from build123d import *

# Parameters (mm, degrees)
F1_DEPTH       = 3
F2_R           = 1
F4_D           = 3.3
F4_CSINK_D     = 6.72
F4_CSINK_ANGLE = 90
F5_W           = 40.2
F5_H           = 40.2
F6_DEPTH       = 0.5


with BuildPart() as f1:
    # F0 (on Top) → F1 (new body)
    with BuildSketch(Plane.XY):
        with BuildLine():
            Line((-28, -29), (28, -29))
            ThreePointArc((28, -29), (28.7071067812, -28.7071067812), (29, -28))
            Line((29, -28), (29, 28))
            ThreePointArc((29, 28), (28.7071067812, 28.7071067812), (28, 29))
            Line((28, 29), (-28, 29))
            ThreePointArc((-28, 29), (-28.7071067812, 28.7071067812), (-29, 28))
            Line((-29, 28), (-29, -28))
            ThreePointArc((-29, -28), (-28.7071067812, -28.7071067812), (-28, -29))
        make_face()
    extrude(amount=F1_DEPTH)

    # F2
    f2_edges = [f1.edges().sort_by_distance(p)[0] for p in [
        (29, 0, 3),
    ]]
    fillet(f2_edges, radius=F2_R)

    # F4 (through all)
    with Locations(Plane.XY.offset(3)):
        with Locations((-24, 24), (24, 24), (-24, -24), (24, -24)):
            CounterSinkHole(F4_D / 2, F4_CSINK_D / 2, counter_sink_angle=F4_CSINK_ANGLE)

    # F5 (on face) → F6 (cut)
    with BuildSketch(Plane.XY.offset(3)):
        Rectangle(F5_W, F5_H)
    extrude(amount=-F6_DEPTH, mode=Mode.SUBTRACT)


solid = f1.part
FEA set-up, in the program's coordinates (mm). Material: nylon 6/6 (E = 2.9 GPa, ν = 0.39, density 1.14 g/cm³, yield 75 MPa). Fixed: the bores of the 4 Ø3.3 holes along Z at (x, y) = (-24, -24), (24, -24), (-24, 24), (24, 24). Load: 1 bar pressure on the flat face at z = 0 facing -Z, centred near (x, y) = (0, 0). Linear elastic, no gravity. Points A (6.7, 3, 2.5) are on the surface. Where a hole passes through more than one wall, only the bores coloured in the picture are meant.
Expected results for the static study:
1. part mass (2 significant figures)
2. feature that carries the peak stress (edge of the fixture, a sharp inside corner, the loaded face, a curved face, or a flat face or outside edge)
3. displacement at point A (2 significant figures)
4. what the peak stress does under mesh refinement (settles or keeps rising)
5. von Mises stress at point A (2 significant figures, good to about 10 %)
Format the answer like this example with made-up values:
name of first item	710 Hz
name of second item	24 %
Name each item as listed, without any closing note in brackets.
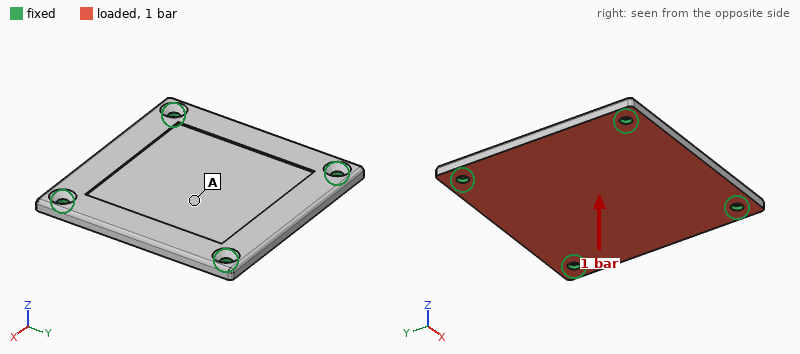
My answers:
part mass	10 g
feature that carries the peak stress	edge of the fixture
displacement at point A	0.84 mm
what the peak stress does under mesh refinement	keeps rising
von Mises stress at point A	12 MPa
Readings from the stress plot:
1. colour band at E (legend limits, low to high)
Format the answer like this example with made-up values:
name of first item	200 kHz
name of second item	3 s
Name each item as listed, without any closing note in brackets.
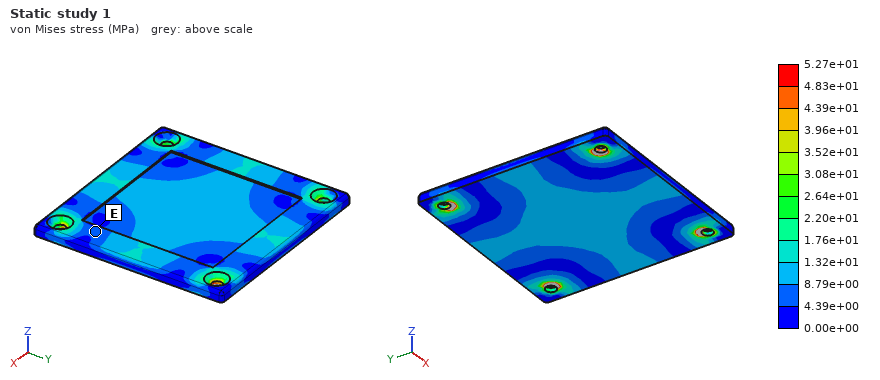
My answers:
colour band at E	4.39e+00 to 8.79e+00 MPa
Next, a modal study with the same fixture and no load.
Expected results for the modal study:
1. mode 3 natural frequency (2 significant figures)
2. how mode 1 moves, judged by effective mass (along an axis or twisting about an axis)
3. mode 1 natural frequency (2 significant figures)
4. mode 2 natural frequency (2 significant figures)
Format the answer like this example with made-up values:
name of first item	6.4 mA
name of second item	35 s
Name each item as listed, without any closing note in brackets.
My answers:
mode 3 natural frequency	2000 Hz
how mode 1 moves, judged by effective mass	along Z
mode 1 natural frequency	1200 Hz
mode 2 natural frequency	2000 Hz
